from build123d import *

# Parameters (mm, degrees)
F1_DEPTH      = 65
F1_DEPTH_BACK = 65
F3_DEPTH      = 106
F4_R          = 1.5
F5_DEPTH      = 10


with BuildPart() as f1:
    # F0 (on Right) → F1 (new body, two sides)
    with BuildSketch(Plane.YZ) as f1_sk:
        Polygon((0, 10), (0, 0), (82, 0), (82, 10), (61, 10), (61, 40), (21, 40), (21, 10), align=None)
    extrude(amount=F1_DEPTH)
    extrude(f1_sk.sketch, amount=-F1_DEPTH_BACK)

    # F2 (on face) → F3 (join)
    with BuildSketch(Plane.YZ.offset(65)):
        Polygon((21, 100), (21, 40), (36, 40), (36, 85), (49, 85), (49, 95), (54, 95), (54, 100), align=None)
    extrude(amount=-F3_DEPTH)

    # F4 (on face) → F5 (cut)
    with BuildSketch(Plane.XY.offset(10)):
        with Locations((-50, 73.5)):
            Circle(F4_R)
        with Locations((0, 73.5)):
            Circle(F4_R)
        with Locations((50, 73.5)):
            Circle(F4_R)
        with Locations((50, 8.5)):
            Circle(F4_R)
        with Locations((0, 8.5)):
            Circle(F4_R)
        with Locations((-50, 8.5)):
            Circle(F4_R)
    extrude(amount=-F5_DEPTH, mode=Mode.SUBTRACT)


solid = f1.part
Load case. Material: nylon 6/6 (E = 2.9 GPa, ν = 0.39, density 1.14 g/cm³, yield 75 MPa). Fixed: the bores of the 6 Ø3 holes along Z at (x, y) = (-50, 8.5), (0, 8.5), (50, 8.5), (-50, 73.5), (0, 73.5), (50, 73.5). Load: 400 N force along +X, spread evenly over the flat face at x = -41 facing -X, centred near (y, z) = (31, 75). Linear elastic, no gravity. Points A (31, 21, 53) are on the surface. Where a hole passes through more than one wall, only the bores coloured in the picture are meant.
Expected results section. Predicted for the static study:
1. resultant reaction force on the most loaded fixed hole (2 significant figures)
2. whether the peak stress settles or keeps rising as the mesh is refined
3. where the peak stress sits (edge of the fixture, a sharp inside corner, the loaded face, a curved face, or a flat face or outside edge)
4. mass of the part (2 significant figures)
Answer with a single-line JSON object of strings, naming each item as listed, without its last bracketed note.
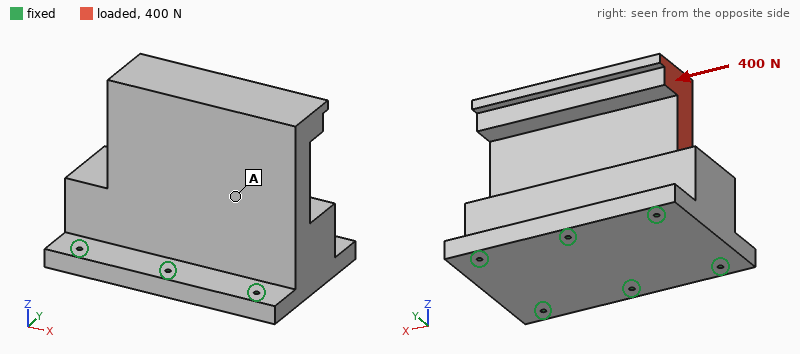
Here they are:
{"resultant reaction force on the most loaded fixed hole": "170 N", "whether the peak stress settles or keeps rising as the mesh is refined": "keeps rising", "where the peak stress sits": "edge of the fixture", "mass of the part": "430 g"}
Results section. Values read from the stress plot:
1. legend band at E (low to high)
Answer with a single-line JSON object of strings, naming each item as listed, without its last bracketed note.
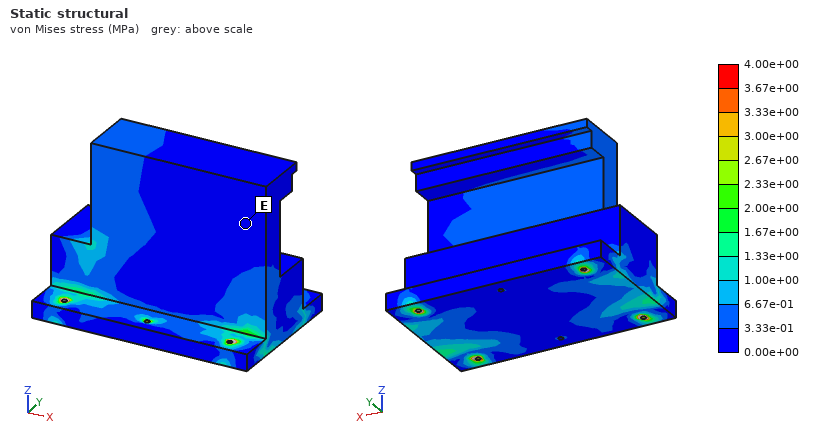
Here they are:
{"legend band at E": "0.00e+00 to 3.33e-01 MPa"}
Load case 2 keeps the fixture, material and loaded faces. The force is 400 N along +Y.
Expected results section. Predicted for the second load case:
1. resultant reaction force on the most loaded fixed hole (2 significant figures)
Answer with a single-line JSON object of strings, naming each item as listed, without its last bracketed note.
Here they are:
{"resultant reaction force on the most loaded fixed hole": "220 N"}
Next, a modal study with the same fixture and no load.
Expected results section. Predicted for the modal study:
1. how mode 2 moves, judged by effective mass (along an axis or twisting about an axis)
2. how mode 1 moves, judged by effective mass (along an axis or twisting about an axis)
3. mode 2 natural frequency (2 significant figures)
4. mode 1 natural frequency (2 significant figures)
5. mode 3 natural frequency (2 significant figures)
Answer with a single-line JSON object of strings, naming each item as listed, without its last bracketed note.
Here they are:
{"how mode 2 moves, judged by effective mass": "along X", "how mode 1 moves, judged by effective mass": "along Y", "mode 2 natural frequency": "910 Hz", "mode 1 natural frequency": "550 Hz", "mode 3 natural frequency": "1100 Hz"}
